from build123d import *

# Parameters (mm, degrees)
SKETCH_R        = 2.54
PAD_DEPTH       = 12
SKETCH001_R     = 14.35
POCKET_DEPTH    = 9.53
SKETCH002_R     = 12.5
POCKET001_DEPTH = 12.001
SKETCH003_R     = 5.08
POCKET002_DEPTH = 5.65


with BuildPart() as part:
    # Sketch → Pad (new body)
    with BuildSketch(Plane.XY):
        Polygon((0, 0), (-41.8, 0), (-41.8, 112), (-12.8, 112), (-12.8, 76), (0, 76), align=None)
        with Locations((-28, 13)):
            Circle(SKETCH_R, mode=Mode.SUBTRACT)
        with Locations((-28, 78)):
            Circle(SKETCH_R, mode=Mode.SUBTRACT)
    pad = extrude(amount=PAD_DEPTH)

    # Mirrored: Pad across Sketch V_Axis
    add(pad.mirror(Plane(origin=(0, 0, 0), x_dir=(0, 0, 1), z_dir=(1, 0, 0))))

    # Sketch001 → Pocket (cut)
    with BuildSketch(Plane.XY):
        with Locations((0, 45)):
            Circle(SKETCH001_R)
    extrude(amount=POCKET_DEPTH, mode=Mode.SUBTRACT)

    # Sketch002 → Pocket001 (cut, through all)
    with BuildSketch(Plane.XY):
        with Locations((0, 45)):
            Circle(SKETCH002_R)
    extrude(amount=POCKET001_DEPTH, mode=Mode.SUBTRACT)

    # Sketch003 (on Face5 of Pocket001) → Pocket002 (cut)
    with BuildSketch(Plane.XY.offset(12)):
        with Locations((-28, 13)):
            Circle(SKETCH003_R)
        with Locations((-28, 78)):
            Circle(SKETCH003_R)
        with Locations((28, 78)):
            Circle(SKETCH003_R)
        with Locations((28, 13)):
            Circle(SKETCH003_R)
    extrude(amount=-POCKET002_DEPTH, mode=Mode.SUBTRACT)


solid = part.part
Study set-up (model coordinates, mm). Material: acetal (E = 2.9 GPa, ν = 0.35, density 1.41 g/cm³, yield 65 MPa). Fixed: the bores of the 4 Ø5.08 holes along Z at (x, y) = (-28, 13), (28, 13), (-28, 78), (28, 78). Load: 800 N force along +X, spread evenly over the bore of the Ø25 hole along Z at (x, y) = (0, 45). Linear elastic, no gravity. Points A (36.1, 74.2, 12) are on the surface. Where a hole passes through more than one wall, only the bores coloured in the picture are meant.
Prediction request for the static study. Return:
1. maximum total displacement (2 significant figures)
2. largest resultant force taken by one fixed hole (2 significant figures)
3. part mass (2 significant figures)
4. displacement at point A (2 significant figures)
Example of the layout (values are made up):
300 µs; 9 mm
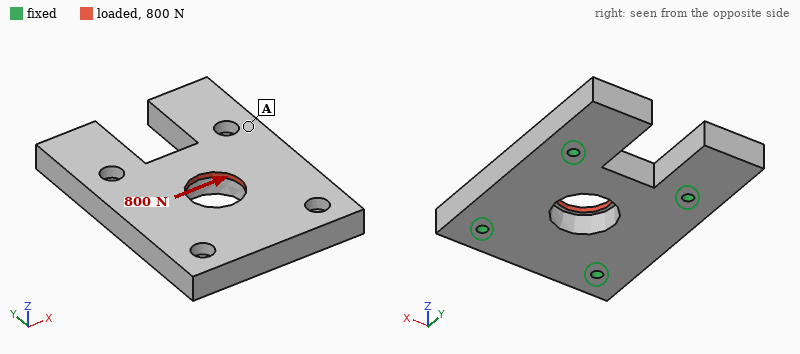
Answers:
36 µm; 240 N; 130 g; 11 µm
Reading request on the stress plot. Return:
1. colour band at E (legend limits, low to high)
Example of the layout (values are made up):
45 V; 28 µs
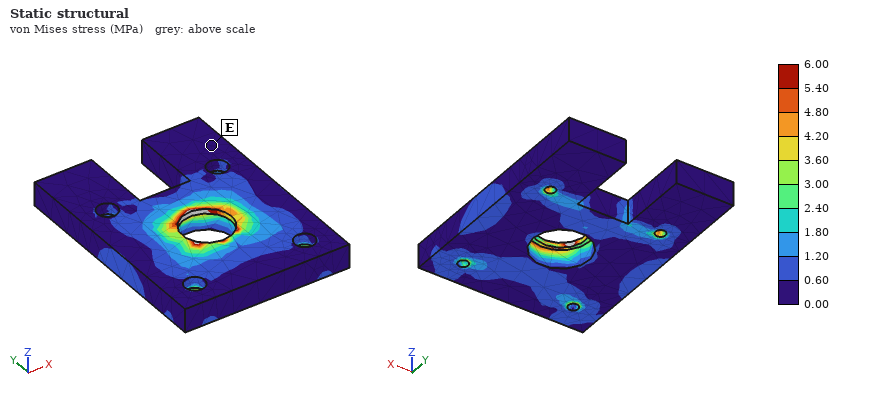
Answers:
0.00 to 0.60 MPa
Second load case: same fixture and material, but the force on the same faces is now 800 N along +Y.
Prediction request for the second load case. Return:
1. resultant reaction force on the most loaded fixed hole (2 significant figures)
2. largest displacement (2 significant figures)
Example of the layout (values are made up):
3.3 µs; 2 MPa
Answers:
230 N; 34 µm
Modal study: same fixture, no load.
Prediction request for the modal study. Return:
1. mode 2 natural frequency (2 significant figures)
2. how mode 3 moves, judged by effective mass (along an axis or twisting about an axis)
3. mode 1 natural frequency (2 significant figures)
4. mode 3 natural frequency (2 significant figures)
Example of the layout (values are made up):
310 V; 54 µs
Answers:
1600 Hz; along Z; 1500 Hz; 2300 Hz
